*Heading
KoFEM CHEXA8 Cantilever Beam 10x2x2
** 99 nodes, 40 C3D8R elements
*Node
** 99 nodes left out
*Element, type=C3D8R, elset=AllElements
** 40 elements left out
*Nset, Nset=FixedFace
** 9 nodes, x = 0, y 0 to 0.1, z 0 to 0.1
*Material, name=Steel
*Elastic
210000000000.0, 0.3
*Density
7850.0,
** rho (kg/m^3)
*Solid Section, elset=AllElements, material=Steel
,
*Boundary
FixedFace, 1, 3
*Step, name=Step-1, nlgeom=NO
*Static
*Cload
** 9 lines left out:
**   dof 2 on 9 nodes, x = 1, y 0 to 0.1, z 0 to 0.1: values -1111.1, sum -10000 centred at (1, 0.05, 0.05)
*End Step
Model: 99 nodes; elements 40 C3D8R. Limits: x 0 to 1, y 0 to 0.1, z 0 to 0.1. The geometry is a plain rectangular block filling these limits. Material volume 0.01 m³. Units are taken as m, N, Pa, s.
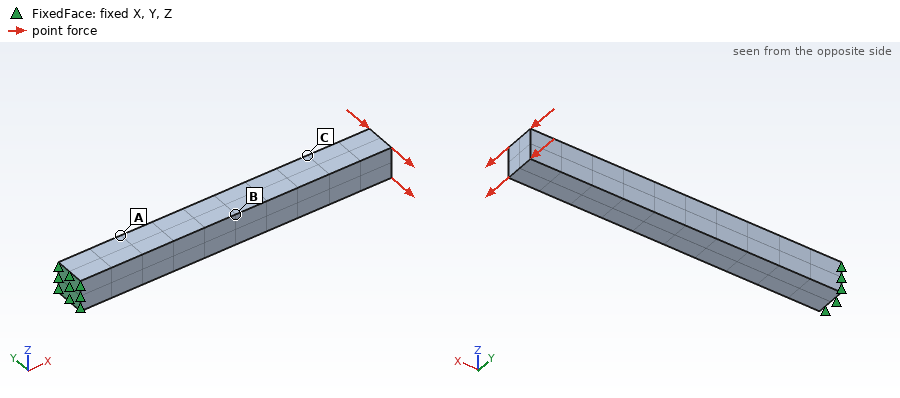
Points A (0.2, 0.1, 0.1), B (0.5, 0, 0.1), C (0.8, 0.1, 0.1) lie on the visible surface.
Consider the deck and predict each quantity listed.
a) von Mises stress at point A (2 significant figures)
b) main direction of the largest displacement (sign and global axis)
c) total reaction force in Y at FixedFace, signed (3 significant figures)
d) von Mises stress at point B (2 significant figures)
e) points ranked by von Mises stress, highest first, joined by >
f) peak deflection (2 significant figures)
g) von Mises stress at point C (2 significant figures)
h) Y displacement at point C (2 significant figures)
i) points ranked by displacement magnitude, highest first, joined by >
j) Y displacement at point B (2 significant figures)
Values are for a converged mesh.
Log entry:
4.8e+07 Pa
-Y
10000 N
3.0e+07 Pa
A > B > C
0.0019 m
1.2e+07 Pa
-0.0013 m
C > B > A
-5.9e-04 m
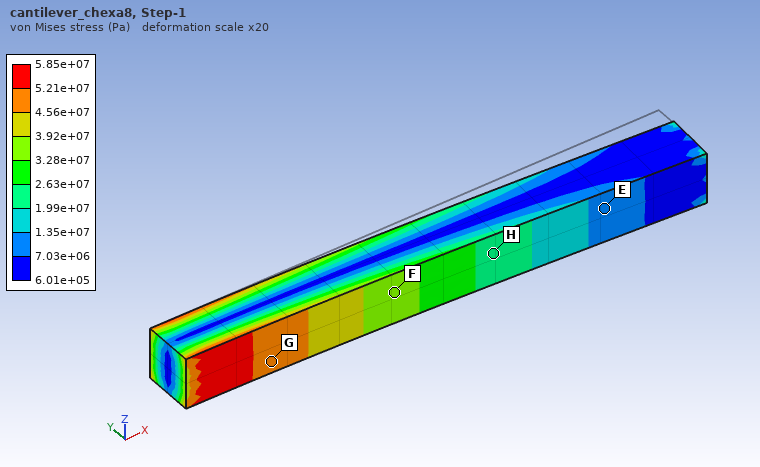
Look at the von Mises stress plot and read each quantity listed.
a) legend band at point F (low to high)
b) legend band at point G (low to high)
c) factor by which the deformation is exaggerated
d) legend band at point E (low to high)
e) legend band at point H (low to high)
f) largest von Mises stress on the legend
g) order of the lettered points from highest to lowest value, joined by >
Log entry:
3.28e+07 to 3.92e+07 Pa
4.56e+07 to 5.21e+07 Pa
20
7.03e+06 to 1.35e+07 Pa
1.99e+07 to 2.63e+07 Pa
5.85e+07 Pa
G > F > H > E
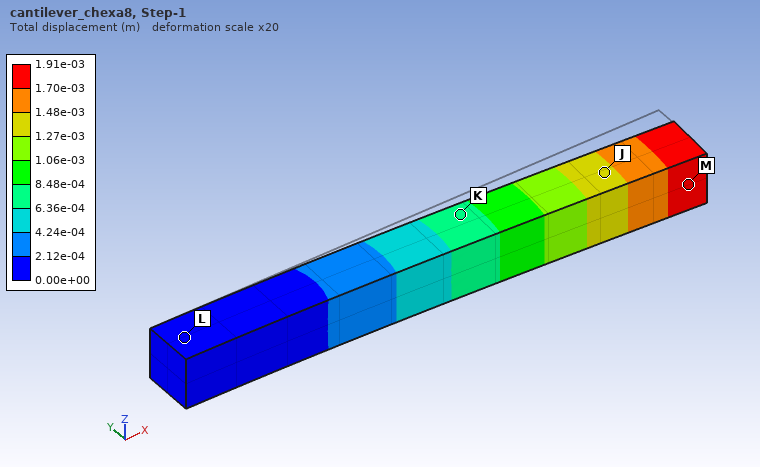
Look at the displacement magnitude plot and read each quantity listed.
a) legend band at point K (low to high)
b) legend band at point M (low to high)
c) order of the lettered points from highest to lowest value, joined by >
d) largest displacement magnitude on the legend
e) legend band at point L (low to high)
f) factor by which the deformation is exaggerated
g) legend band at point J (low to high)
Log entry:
6.36e-04 to 8.48e-04 m
1.70e-03 to 1.91e-03 m
M > J > K > L
1.91e-03 m
0.00e+00 to 2.12e-04 m
20
1.27e-03 to 1.48e-03 m
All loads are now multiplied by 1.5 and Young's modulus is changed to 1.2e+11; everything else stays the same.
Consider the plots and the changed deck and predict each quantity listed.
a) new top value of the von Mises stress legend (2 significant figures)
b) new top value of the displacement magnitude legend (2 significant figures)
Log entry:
8.8e+07 Pa
0.0050 m
